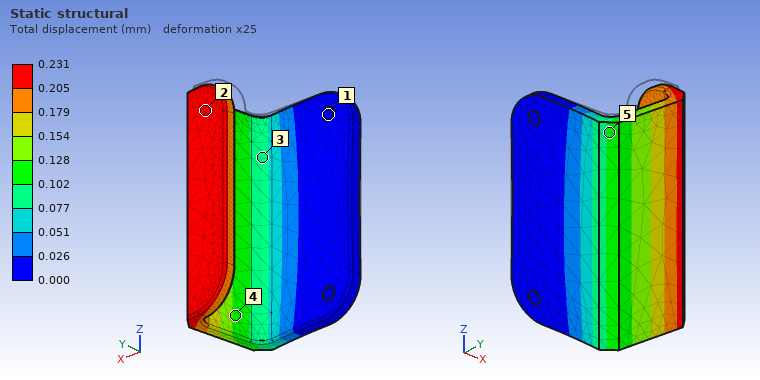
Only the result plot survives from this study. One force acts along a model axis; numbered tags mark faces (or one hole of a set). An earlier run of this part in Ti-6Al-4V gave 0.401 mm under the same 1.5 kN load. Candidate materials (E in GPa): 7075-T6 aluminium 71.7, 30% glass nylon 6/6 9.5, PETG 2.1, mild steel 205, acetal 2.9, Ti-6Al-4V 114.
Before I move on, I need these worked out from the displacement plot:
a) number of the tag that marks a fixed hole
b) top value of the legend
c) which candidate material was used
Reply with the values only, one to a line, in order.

1
0.231 mm
mild steel
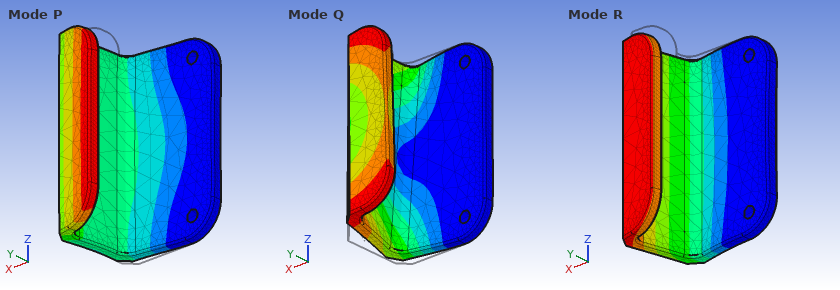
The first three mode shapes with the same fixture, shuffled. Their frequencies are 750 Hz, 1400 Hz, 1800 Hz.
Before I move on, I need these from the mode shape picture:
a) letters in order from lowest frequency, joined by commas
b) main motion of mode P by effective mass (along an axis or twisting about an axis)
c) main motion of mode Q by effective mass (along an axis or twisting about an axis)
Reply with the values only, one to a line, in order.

R, Q, P
along Y
along Z
